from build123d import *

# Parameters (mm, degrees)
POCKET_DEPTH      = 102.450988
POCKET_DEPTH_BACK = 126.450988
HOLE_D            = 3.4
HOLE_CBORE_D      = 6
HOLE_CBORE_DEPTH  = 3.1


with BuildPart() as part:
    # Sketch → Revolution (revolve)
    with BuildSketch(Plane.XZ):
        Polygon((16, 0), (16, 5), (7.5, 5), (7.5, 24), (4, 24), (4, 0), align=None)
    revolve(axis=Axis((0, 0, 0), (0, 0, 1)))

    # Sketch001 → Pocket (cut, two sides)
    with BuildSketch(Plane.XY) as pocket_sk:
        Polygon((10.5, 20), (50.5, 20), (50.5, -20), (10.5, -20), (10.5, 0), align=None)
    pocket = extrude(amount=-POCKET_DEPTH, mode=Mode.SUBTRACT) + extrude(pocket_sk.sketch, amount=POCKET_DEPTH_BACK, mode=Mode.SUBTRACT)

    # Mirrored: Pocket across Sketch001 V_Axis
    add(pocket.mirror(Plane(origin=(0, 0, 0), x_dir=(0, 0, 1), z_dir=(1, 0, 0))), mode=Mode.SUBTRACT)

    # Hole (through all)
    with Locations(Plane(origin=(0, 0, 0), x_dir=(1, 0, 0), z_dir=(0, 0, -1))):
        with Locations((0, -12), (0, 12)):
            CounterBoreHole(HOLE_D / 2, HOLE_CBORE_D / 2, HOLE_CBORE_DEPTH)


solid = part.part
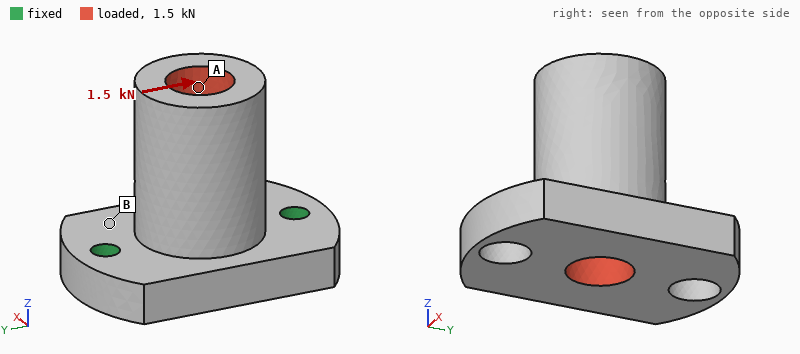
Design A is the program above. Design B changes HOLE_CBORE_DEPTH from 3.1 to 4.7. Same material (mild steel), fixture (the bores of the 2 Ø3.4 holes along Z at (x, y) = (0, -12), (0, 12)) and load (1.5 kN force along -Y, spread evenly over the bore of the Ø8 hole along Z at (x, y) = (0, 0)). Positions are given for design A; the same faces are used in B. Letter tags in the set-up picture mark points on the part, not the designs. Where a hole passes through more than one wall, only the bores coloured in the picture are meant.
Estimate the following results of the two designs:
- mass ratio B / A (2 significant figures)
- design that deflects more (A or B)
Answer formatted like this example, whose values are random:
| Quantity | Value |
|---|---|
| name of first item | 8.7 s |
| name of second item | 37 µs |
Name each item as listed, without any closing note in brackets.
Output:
| Quantity | Value |
|---|---|
| mass ratio B / A | 0.99 |
| design that deflects more | B |
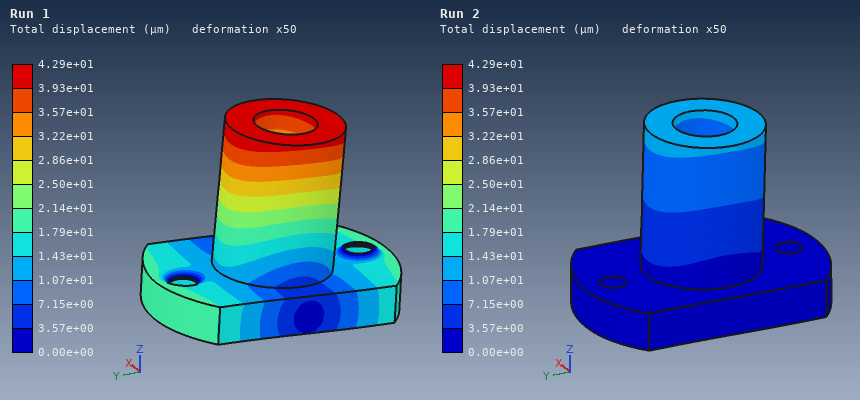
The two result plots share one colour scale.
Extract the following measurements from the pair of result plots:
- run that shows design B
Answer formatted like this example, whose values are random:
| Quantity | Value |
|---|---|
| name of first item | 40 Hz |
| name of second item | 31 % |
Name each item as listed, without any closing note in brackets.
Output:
| Quantity | Value |
|---|---|
| run that shows design B | Run 1 |
